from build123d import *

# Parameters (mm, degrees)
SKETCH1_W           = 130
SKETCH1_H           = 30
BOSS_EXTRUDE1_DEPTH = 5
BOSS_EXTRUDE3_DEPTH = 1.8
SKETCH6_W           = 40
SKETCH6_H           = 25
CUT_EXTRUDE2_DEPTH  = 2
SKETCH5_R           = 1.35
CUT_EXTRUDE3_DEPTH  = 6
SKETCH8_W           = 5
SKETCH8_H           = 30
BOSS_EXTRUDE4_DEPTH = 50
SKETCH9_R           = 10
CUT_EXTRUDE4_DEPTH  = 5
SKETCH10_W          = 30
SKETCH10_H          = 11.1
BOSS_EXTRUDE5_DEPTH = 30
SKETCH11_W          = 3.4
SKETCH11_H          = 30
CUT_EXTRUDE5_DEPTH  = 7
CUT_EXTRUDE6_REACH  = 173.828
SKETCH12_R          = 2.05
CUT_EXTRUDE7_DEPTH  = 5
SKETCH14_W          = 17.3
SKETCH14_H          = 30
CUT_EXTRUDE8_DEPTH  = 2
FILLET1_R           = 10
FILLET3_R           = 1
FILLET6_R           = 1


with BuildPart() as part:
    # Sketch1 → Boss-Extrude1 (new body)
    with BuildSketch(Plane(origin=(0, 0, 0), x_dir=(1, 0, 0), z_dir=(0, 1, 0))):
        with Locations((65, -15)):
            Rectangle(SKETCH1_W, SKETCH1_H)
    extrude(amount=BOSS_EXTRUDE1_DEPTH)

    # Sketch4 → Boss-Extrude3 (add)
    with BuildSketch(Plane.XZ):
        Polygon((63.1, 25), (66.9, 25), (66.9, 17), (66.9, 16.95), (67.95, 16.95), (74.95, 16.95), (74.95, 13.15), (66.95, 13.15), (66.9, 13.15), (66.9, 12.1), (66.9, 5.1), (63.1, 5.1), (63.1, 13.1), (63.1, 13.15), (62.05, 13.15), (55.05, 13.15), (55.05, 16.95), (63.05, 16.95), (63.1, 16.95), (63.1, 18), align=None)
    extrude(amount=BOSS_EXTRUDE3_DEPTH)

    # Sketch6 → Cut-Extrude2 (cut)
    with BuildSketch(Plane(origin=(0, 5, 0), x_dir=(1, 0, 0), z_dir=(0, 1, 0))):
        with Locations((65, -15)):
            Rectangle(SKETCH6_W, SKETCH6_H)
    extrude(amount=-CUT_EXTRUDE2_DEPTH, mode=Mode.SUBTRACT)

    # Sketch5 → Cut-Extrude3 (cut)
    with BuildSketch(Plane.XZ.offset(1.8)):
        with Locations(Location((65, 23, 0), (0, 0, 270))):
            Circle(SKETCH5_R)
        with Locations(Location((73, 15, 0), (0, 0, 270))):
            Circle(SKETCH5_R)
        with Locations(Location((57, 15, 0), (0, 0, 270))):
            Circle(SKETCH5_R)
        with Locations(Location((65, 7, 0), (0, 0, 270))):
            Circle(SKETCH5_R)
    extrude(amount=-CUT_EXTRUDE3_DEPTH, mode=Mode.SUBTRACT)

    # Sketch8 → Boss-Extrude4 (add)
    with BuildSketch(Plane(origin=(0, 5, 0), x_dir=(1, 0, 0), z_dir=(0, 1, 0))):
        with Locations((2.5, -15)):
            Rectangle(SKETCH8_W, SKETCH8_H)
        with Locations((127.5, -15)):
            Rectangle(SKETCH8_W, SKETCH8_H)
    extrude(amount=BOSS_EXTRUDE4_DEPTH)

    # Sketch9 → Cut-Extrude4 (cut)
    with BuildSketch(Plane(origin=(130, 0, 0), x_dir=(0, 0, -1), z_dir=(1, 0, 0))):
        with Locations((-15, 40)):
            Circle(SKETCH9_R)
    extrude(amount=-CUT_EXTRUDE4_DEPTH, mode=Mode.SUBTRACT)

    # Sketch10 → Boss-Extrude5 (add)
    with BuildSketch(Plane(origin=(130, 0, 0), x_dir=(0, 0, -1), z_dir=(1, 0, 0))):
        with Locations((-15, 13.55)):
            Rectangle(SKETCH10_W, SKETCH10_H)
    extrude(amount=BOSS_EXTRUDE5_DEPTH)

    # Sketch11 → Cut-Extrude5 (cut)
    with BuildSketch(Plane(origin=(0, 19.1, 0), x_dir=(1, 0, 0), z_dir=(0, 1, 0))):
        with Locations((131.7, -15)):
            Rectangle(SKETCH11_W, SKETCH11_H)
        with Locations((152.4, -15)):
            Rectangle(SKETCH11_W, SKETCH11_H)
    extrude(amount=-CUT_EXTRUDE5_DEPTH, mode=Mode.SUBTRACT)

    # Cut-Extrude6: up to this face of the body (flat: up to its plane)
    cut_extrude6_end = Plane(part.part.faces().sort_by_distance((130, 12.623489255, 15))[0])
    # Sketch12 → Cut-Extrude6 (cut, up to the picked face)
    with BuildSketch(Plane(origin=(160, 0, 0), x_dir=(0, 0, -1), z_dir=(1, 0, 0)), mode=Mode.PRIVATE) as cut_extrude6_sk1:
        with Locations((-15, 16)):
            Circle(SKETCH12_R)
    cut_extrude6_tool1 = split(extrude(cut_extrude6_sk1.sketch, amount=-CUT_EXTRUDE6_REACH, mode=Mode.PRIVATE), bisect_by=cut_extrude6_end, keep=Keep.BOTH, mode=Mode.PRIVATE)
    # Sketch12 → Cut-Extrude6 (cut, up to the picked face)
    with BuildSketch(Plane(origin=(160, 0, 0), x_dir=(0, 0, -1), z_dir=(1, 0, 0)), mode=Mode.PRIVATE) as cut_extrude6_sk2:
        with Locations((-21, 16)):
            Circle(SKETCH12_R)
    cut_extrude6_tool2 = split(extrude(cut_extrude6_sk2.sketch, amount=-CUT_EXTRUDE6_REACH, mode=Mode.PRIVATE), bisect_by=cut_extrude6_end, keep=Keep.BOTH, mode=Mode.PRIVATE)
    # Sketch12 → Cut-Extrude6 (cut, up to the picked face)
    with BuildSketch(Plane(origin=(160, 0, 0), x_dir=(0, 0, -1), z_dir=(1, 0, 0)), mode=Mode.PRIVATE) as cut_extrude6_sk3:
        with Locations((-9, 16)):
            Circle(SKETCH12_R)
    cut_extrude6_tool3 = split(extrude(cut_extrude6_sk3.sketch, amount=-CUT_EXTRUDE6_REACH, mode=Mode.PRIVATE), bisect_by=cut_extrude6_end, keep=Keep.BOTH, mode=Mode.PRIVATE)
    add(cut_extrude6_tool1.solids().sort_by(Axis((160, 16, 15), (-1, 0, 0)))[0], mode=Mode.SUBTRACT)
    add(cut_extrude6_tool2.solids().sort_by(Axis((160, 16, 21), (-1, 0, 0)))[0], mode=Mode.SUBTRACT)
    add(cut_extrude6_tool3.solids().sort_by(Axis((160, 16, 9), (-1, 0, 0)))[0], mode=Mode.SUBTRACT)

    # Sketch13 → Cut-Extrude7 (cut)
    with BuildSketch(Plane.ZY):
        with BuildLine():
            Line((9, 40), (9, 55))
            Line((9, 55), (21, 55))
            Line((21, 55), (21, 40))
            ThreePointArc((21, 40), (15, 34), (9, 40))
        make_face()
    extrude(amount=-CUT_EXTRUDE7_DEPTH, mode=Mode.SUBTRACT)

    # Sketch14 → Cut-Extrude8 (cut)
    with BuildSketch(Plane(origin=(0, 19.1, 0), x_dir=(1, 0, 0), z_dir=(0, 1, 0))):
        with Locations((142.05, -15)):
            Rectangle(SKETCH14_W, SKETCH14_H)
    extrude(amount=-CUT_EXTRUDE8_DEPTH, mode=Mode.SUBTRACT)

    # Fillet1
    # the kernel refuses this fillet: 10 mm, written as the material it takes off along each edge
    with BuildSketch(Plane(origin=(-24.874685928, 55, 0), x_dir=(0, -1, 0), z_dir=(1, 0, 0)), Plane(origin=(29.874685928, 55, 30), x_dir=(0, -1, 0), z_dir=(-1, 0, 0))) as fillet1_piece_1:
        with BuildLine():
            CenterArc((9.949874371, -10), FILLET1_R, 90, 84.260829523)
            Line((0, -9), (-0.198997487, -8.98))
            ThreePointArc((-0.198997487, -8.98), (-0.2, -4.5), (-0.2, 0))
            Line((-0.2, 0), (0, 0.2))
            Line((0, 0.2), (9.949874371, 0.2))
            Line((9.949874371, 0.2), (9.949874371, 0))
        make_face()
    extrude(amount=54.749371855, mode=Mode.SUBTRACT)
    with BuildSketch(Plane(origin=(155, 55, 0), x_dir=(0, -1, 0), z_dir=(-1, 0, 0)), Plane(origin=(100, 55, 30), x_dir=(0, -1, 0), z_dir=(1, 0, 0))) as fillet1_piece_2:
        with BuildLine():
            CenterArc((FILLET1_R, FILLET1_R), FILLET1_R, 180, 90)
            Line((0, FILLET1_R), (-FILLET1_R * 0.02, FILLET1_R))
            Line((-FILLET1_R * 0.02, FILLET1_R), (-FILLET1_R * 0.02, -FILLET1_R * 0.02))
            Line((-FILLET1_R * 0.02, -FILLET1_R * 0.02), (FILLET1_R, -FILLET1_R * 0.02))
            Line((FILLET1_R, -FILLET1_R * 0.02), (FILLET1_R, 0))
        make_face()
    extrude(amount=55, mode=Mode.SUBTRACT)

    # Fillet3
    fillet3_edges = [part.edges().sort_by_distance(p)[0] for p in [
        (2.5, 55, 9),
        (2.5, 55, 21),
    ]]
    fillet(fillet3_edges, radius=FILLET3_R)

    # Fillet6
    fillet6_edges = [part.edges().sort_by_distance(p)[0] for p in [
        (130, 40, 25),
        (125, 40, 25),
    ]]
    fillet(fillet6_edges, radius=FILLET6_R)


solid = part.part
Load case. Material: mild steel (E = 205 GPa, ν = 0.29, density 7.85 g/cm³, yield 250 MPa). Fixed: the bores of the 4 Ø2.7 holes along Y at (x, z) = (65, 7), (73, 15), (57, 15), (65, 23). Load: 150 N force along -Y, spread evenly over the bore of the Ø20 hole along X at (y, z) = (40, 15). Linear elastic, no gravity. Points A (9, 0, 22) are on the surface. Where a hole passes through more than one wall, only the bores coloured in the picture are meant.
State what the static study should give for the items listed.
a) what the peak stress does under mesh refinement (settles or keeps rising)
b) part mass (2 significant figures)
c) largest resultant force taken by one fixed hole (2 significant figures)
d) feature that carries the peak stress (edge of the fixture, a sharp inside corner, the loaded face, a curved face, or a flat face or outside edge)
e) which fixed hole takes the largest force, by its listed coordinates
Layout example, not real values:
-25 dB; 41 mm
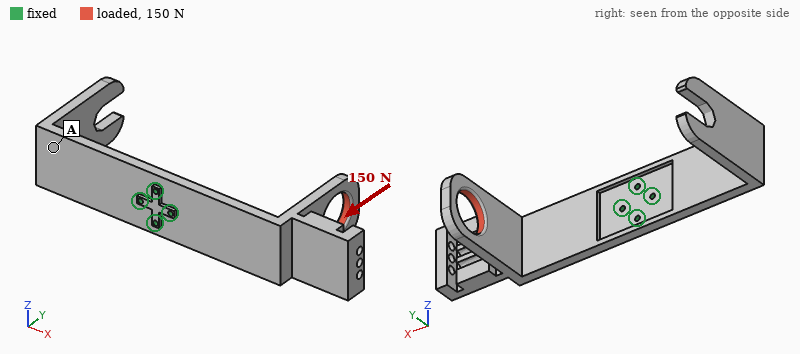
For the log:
keeps rising; 280 g; 670 N; edge of the fixture; (73, 15)
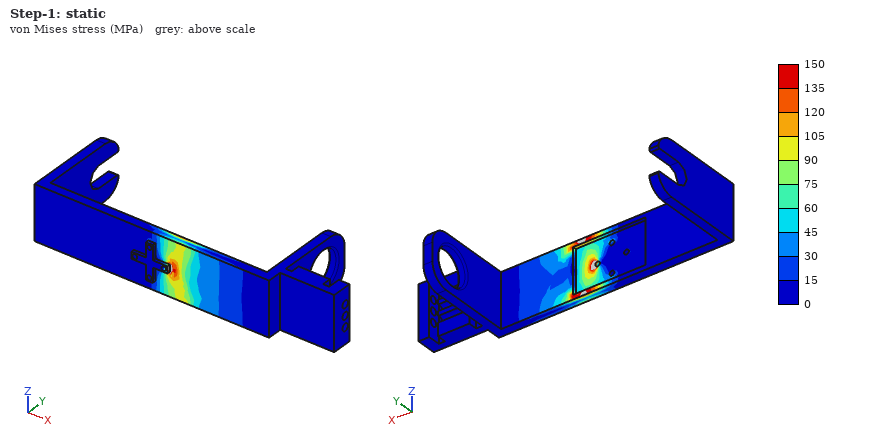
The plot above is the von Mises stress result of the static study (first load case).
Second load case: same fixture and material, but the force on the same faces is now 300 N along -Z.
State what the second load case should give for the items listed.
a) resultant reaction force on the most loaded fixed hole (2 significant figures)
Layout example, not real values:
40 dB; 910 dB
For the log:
800 N
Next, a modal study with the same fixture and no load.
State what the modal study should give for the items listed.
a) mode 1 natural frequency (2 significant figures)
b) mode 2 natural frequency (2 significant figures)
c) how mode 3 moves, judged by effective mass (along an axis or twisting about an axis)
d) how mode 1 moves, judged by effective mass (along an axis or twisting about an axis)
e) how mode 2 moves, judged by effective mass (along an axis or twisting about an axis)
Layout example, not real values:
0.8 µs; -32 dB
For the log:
260 Hz; 390 Hz; along Z; along Y; along Y
